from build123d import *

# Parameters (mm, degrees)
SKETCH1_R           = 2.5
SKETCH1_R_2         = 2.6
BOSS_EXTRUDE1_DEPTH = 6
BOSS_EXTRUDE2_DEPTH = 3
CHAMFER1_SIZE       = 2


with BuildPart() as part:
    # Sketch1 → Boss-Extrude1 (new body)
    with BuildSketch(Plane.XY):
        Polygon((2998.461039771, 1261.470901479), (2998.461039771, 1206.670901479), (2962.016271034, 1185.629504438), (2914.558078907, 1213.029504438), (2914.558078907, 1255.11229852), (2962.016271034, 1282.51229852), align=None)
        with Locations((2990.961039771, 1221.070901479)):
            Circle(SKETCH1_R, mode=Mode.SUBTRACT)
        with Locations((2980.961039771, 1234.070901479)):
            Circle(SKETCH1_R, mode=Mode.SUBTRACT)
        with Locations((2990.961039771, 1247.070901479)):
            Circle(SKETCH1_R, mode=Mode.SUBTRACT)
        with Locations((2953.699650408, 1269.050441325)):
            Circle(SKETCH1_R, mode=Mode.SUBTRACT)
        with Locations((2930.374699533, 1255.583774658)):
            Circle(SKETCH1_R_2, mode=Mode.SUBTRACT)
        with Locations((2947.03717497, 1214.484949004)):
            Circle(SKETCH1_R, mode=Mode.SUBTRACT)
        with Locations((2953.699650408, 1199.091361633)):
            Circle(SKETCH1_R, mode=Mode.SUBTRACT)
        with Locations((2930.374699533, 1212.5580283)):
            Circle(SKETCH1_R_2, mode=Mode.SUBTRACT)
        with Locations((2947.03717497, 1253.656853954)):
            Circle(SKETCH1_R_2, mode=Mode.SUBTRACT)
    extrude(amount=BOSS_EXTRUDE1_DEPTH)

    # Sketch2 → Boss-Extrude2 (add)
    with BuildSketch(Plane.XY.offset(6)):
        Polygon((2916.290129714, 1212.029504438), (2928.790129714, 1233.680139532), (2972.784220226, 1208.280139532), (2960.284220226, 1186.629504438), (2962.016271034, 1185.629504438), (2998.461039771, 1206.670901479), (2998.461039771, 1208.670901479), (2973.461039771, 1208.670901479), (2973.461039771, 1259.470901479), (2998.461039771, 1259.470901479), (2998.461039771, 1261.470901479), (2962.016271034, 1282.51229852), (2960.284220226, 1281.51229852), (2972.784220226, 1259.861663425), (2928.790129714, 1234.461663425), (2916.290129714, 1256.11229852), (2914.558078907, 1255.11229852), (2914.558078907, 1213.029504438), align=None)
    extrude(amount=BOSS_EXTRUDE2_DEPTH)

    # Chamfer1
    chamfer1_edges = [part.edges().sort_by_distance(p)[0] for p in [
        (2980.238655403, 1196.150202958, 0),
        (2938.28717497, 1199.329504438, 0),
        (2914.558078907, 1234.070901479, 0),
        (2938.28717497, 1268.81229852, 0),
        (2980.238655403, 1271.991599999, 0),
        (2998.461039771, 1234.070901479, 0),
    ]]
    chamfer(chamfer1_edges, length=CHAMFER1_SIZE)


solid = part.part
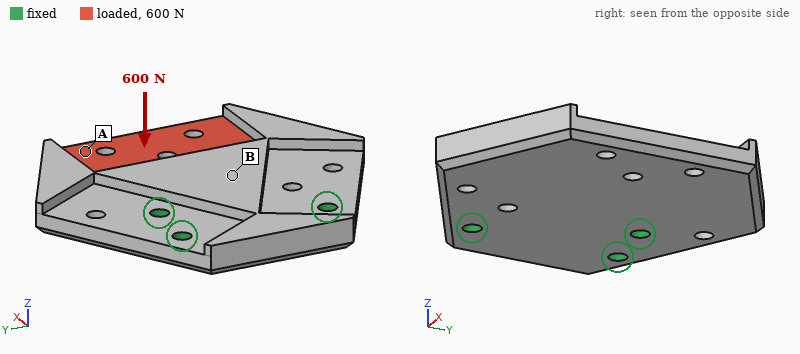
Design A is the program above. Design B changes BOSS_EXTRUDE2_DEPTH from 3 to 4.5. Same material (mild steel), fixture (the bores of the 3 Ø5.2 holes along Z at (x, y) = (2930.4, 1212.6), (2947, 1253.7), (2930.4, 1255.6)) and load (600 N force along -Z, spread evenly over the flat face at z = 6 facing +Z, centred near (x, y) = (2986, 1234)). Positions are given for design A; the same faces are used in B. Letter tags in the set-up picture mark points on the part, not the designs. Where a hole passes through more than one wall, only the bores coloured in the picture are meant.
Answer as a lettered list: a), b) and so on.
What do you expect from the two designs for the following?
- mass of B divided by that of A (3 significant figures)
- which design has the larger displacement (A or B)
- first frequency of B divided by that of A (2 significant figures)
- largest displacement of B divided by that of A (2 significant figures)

a) 1.08
b) A
c) 1.0
d) 0.86
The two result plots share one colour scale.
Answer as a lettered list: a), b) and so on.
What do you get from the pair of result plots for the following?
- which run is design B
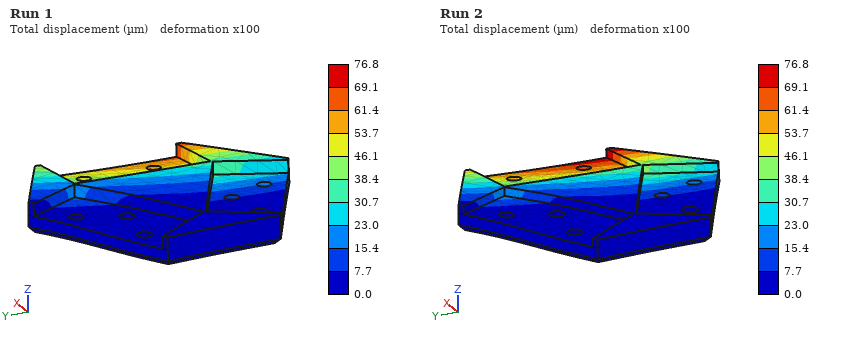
a) Run 1
